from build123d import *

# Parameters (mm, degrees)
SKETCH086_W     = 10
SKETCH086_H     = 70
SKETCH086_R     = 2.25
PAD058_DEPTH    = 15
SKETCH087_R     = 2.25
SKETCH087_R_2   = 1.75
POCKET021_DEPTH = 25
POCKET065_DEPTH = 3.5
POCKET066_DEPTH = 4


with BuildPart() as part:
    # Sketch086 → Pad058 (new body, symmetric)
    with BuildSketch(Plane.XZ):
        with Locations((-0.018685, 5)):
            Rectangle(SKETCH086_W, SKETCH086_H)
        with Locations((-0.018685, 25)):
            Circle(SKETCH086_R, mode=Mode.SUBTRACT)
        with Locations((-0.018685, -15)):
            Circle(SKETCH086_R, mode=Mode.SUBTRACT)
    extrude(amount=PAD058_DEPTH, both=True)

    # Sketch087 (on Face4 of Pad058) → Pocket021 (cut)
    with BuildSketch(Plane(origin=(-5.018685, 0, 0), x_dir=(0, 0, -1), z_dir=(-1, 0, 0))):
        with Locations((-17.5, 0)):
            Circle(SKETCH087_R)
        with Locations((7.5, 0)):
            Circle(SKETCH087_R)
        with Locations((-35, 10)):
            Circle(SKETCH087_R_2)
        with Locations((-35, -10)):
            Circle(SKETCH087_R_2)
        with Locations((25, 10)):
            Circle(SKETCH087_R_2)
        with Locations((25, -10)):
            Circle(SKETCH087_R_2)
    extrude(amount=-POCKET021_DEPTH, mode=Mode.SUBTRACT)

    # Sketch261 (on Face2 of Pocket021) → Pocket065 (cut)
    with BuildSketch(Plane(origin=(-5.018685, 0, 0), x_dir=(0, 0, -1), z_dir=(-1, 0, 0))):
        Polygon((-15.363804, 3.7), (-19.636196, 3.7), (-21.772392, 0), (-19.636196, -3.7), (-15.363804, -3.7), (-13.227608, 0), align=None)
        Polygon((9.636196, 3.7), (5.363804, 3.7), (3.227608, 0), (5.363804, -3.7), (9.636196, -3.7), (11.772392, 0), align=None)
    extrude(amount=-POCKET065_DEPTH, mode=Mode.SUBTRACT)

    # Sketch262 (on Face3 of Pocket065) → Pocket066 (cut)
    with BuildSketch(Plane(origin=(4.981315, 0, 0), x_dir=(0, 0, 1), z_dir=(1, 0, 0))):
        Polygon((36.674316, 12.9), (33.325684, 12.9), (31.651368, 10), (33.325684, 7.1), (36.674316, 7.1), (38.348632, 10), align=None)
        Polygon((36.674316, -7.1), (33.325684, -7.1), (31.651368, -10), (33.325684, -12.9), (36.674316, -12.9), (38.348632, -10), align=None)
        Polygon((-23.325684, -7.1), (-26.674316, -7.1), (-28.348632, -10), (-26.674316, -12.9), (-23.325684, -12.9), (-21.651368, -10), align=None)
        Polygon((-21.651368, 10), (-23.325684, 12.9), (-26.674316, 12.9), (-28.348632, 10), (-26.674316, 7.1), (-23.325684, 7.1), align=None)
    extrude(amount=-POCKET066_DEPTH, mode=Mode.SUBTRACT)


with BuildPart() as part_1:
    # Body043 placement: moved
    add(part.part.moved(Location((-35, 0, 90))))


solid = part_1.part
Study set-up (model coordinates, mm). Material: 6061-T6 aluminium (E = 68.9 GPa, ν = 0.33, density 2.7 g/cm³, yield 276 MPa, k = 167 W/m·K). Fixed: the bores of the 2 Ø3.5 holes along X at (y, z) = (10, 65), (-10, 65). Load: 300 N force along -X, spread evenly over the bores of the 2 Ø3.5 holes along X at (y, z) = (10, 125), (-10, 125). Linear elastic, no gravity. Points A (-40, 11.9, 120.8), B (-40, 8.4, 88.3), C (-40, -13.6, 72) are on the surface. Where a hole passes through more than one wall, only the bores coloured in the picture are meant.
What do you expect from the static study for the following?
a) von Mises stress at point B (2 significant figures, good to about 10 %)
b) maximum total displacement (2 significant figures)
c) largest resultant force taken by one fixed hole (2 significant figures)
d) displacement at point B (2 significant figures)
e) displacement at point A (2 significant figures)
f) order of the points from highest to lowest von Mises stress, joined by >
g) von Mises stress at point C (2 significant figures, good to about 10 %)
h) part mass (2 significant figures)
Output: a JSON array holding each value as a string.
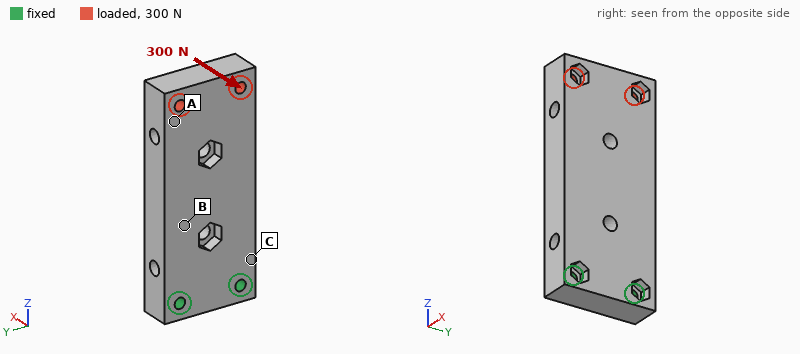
["26 MPa", "0.24 mm", "160 N", "0.057 mm", "0.19 mm", "C > B > A", "43 MPa", "51 g"]
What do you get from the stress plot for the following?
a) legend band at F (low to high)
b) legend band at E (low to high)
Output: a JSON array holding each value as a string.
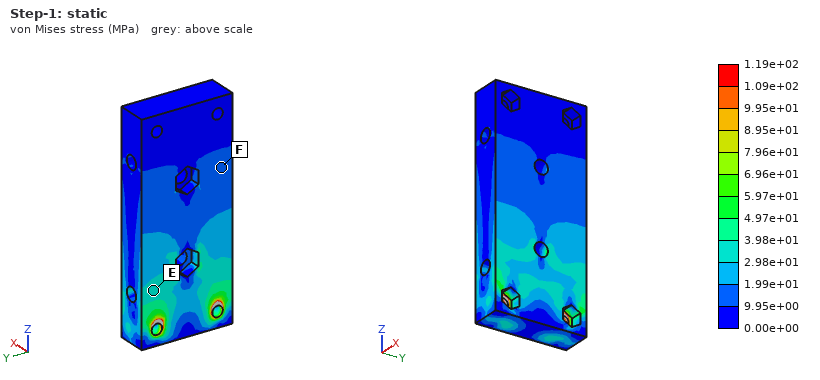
["9.95e+00 to 1.99e+01 MPa", "2.98e+01 to 3.98e+01 MPa"]
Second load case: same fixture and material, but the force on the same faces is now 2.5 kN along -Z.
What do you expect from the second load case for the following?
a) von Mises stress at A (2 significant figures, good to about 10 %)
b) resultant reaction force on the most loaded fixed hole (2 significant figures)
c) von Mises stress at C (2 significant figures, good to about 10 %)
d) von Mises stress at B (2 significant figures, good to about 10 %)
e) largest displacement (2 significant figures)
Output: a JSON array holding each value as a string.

["28 MPa", "1.3 kN", "25 MPa", "22 MPa", "68 µm"]
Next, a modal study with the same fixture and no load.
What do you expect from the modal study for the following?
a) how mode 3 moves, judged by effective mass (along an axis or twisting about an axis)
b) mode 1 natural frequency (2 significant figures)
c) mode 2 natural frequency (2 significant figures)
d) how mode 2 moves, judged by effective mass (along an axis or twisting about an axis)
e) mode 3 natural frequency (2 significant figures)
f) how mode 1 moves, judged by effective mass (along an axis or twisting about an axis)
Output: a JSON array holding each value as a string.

["twisting about Z", "1500 Hz", "4300 Hz", "along Y", "6800 Hz", "along X"]
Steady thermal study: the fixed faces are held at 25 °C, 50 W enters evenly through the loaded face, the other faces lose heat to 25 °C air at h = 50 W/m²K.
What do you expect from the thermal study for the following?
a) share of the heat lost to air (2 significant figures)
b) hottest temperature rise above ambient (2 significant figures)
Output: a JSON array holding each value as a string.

["23 %", "68 K"]
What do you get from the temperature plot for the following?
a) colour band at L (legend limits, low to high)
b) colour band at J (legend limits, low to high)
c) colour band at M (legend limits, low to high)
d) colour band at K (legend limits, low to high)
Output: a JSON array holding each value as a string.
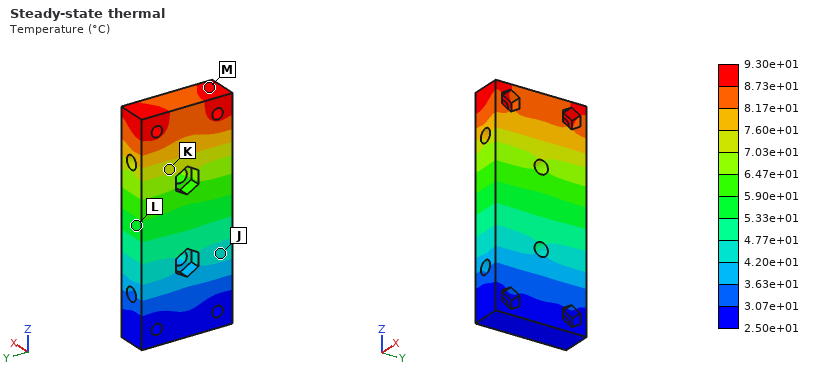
["5.33e+01 to 5.90e+01 °C", "4.20e+01 to 4.77e+01 °C", "8.73e+01 to 9.30e+01 °C", "7.03e+01 to 7.60e+01 °C"]
